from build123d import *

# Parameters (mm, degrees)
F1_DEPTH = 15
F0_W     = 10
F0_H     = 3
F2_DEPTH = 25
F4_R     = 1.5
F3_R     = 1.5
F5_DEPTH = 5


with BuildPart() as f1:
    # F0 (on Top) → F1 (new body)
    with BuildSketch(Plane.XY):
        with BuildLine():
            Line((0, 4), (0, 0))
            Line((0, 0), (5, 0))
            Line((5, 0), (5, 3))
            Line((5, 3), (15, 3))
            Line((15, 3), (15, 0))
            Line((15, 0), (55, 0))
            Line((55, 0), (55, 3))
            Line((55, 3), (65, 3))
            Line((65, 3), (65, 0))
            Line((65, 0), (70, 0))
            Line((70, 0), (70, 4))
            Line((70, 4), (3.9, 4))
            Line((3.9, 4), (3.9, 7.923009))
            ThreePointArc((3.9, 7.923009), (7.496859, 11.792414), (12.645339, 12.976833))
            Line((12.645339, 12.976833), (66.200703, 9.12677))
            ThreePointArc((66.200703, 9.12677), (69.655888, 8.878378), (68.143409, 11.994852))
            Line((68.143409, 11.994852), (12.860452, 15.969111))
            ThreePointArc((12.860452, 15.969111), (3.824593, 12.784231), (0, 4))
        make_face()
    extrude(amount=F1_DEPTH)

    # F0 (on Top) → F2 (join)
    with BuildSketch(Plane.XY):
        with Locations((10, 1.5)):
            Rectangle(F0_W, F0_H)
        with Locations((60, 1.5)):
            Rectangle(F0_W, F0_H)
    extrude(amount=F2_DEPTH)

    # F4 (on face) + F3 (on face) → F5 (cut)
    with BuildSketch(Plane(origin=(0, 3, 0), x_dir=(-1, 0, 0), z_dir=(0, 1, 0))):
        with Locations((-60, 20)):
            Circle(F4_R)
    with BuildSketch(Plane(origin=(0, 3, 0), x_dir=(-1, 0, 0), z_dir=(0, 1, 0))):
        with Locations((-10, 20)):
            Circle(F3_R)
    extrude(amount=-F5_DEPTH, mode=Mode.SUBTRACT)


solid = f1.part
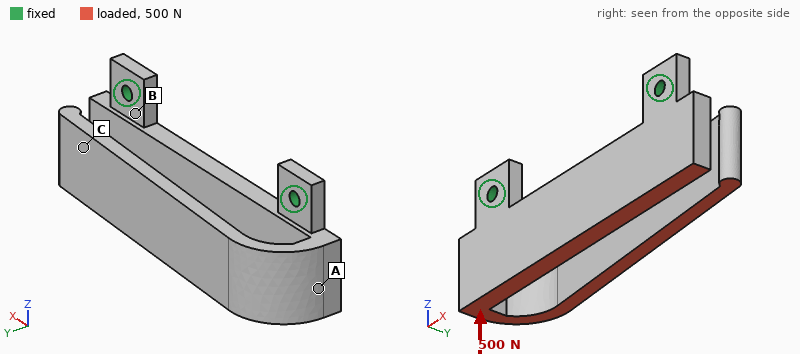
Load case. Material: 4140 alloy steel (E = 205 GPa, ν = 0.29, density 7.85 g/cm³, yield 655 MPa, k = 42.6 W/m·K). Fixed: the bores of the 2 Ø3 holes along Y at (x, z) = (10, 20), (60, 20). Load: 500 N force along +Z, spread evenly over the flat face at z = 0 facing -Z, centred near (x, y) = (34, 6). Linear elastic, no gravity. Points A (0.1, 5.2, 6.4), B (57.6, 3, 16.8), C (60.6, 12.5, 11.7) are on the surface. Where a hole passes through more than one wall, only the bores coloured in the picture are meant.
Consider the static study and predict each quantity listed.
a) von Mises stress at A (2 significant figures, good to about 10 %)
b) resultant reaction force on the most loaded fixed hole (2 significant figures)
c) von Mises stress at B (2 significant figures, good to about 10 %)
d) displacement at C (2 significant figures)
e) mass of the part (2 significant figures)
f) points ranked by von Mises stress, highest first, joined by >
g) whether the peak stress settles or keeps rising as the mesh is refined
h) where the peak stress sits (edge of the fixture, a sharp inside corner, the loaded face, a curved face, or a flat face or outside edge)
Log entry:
150 MPa
330 N
59 MPa
0.32 mm
64 g
A > B > C
keeps rising
edge of the fixture
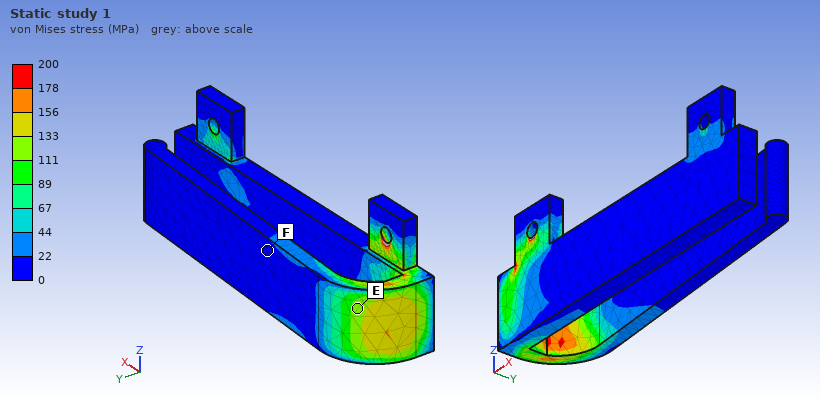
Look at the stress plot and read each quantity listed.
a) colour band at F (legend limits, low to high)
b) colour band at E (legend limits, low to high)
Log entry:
0 to 22 MPa
111 to 133 MPa
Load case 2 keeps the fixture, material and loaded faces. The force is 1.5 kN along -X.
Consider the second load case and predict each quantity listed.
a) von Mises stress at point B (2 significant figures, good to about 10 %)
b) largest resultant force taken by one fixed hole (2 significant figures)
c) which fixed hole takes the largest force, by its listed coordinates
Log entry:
50 MPa
1.0 kN
(60, 20)
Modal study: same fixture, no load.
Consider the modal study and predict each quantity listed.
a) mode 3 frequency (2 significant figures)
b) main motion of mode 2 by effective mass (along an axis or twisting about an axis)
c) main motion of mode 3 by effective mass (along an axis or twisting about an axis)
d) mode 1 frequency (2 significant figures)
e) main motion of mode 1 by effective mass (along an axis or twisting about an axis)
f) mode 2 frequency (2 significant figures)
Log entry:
2200 Hz
along Z
along Y
420 Hz
along Y
920 Hz
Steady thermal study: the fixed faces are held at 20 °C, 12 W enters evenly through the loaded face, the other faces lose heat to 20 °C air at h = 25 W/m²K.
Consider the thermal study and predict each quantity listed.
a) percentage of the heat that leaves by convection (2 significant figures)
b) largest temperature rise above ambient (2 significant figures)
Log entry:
40 %
66 K
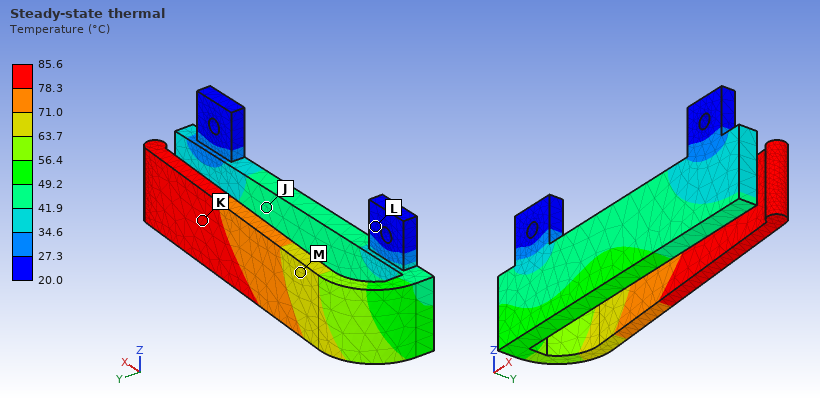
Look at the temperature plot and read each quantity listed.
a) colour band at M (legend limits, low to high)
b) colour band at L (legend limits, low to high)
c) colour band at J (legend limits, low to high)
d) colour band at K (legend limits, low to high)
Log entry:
63.7 to 71.0 °C
20.0 to 27.3 °C
41.9 to 49.2 °C
78.3 to 85.6 °C
